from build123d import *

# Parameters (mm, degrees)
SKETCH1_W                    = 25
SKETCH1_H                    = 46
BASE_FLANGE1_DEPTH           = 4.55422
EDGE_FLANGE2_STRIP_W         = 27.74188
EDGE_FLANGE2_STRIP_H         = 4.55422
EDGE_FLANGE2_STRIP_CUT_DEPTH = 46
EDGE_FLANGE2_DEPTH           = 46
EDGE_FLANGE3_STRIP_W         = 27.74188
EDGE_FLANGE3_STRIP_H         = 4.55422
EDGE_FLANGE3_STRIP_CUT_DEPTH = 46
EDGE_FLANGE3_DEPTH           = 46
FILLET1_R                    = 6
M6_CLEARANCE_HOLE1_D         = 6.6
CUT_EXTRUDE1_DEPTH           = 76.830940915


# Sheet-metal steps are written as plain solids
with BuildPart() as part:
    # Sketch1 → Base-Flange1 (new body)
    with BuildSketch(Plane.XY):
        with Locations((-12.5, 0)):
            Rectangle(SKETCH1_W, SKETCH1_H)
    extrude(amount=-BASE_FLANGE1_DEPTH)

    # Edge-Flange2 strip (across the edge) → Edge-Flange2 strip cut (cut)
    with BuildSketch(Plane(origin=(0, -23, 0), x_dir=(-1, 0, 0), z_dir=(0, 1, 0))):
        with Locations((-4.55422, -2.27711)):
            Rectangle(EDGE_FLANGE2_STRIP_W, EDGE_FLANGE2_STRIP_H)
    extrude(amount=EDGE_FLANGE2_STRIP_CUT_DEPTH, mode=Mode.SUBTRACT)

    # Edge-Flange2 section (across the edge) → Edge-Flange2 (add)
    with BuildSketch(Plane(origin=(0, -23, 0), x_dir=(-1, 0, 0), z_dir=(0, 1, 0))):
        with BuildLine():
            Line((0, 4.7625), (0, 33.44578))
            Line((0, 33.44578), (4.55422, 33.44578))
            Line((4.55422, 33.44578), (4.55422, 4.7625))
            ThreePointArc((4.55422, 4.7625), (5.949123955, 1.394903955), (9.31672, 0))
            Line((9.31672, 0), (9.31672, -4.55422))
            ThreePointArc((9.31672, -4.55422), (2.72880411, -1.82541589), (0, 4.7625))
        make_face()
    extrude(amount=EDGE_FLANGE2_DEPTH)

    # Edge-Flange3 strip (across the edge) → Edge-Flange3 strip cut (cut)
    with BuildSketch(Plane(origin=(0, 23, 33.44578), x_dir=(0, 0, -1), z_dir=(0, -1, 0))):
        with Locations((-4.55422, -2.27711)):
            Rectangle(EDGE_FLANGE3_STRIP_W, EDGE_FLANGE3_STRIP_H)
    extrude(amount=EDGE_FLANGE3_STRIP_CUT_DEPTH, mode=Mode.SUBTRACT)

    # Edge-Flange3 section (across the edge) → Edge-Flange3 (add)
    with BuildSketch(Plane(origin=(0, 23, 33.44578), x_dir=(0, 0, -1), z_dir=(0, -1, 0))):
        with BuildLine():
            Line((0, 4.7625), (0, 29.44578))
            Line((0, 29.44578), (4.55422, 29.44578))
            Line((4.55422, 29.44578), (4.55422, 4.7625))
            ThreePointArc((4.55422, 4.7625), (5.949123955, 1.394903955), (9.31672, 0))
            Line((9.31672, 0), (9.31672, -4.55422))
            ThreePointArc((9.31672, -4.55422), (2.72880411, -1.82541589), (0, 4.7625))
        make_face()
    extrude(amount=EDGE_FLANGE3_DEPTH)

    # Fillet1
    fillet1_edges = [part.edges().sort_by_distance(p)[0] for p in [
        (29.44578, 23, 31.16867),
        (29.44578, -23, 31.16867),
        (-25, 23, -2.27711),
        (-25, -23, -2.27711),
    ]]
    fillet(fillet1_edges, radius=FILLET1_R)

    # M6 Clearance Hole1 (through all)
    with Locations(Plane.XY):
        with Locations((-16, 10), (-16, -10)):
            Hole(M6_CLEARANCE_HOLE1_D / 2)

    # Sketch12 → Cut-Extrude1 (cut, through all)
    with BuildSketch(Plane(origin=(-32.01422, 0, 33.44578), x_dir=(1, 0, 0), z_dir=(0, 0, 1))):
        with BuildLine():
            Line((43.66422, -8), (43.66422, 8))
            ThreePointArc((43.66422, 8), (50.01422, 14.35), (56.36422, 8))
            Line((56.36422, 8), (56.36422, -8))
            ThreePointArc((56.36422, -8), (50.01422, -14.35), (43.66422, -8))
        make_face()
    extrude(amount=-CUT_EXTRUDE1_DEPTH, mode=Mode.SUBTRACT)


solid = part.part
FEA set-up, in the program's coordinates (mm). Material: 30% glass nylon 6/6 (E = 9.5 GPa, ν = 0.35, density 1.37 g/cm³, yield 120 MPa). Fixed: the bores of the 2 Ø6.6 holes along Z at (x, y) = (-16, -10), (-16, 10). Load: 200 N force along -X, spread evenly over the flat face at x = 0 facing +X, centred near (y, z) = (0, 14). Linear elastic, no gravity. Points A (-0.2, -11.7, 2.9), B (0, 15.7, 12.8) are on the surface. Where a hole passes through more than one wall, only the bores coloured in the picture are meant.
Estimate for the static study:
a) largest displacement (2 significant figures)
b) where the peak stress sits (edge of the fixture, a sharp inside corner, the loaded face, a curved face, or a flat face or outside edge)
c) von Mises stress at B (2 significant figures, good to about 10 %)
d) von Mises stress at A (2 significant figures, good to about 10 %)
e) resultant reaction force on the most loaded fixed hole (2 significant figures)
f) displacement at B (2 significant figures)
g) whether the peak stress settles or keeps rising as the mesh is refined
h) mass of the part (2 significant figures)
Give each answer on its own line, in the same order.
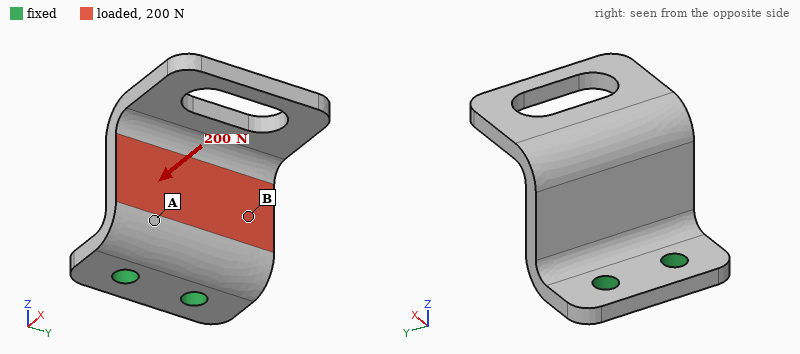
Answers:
0.81 mm
edge of the fixture
4.1 MPa
10 MPa
100 N
0.22 mm
keeps rising
21 g
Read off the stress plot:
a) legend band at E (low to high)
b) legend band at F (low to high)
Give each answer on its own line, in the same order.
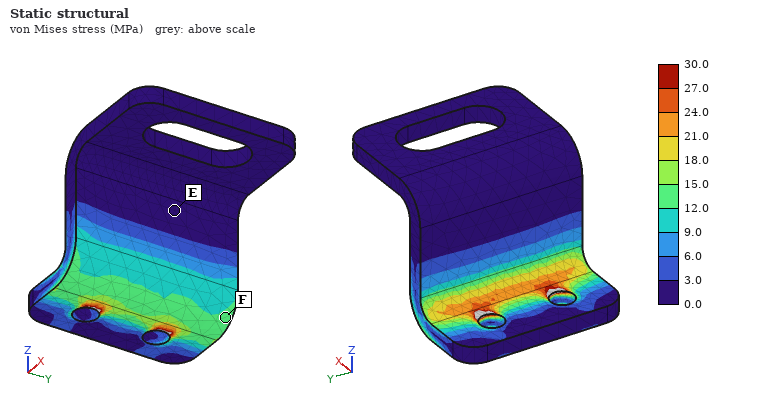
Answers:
0.0 to 3.0 MPa
12.0 to 15.0 MPa
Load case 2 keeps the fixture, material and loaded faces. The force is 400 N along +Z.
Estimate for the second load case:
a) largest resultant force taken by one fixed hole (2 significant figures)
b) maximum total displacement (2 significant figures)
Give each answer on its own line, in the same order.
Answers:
200 N
0.79 mm
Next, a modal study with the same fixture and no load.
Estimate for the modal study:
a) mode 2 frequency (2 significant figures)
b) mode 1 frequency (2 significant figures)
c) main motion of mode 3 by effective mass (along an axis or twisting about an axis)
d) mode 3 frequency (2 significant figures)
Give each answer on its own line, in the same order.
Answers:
1200 Hz
560 Hz
along Y
1800 Hz
